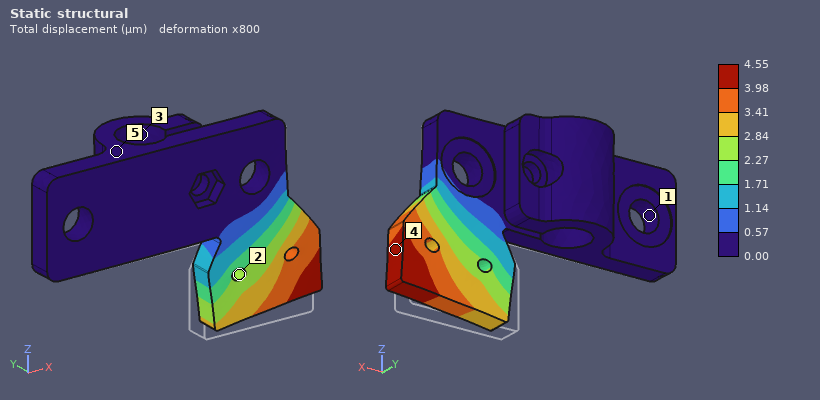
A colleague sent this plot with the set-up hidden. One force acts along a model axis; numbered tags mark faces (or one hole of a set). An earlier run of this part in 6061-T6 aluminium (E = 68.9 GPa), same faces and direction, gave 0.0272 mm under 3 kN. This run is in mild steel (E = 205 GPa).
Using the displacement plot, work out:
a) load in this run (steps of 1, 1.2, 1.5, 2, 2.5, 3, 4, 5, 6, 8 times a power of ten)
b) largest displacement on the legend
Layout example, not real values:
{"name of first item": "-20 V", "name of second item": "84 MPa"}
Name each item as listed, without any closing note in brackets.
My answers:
{"load in this run": "1.5 kN", "largest displacement on the legend": "4.55 µm"}
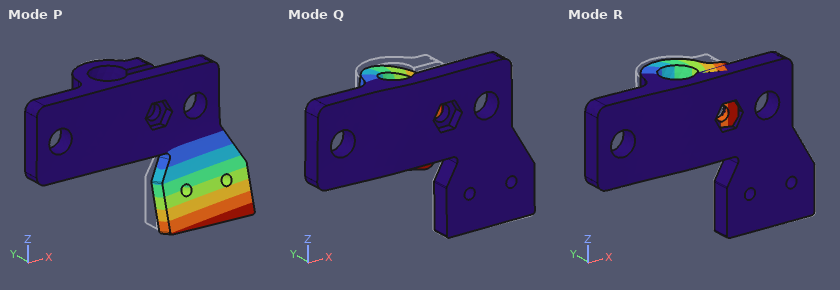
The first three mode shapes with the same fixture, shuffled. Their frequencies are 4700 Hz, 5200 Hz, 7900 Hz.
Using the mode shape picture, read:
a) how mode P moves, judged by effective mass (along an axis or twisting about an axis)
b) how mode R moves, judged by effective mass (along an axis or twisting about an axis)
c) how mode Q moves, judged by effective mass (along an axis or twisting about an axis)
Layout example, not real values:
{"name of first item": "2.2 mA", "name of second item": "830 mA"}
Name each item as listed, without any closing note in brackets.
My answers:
{"how mode P moves, judged by effective mass": "along Y", "how mode R moves, judged by effective mass": "along Y", "how mode Q moves, judged by effective mass": "along Z"}
